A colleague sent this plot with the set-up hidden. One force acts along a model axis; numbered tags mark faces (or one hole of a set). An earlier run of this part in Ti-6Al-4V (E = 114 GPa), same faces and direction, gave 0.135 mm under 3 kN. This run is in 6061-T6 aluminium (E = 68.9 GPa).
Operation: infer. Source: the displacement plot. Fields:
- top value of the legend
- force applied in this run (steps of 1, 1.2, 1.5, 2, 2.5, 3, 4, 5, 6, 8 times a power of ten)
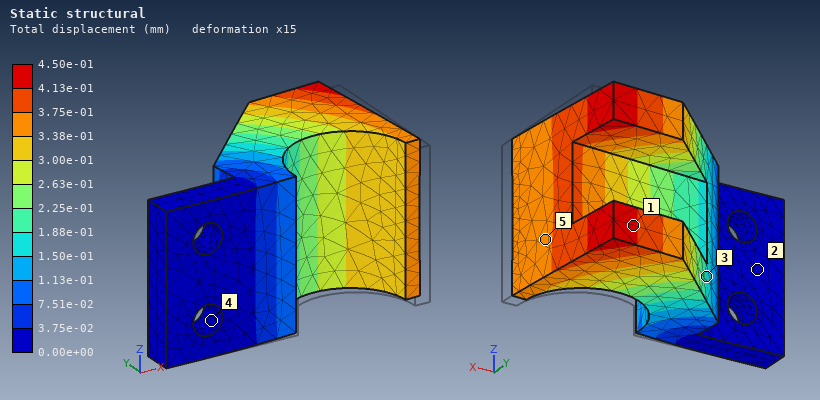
4.50e-01 mm
6 kN
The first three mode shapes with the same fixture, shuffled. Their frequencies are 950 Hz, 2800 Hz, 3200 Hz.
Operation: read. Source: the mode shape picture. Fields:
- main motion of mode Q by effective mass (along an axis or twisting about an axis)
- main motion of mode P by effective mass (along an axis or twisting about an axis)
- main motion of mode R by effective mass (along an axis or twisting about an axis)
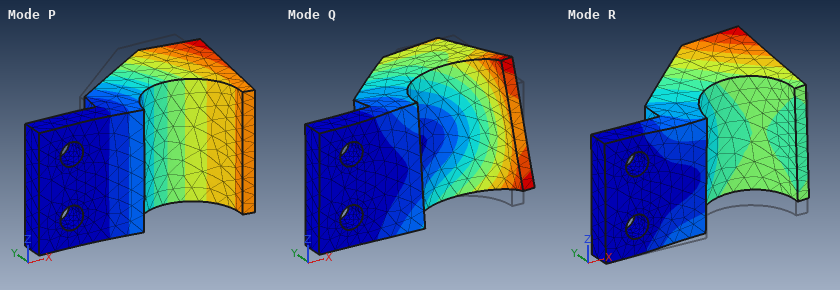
twisting about X
along Y
along Z
